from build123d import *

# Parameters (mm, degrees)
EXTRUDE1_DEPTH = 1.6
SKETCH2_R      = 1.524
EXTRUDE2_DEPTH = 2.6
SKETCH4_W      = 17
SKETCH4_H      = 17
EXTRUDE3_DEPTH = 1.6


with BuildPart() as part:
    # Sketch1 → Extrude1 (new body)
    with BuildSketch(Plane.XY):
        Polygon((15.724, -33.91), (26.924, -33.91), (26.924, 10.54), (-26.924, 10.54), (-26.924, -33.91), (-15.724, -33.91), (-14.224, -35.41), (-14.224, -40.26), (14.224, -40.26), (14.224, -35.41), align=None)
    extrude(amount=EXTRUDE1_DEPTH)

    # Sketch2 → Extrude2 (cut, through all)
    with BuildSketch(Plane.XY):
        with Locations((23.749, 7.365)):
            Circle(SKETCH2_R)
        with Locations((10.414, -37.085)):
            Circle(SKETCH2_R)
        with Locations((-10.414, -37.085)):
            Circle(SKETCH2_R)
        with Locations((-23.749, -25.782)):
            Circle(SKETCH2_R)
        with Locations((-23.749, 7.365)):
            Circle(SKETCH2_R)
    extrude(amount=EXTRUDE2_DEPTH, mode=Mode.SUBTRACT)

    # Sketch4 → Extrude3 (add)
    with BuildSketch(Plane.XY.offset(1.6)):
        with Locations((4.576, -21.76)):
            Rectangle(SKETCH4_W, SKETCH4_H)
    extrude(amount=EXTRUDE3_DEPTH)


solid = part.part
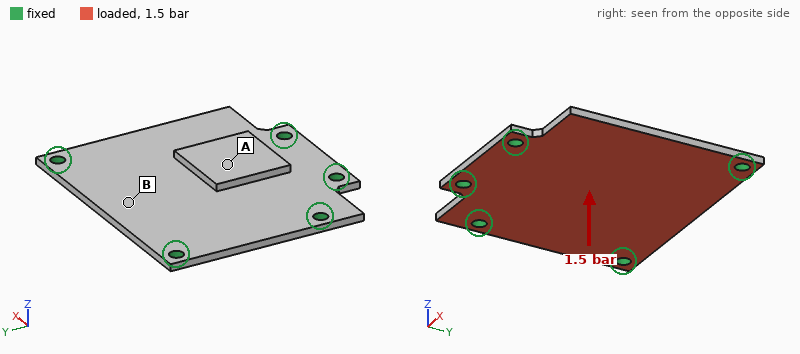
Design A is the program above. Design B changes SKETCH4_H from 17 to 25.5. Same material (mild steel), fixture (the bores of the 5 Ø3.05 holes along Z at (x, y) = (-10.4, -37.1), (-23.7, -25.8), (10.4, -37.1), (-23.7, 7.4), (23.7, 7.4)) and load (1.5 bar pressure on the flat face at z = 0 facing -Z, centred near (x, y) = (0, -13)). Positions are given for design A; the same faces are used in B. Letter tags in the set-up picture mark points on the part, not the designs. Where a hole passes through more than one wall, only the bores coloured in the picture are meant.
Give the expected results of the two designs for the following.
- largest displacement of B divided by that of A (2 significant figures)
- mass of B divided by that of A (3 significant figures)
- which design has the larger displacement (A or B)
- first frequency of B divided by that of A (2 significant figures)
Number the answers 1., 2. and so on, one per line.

1. 0.92
2. 1.05
3. A
4. 1.0
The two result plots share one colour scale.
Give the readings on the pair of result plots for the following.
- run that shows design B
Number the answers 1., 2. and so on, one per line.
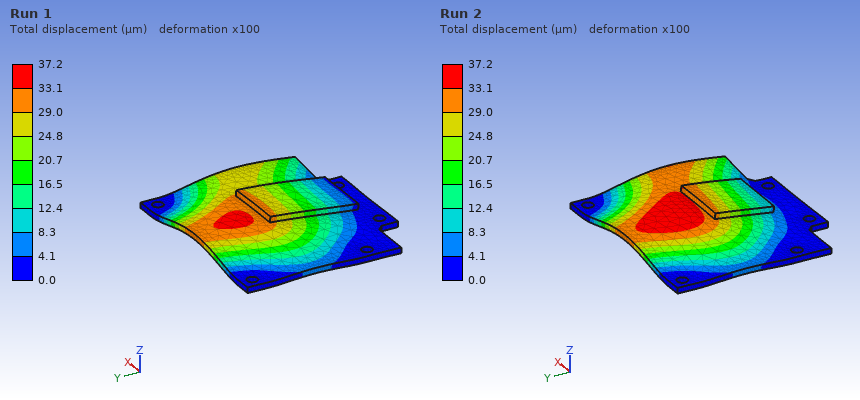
1. Run 1
